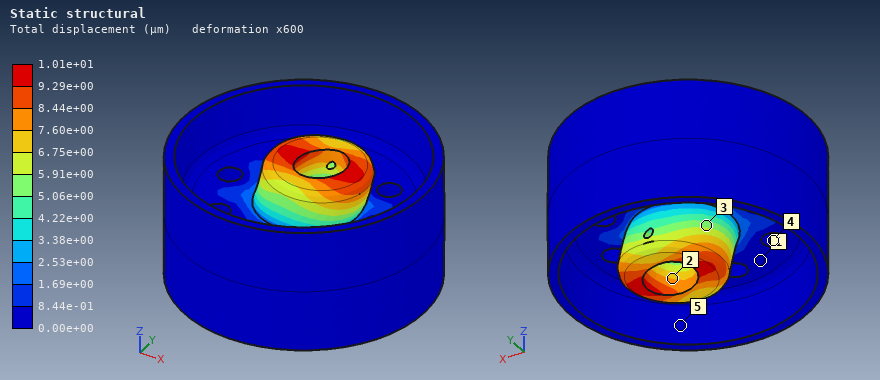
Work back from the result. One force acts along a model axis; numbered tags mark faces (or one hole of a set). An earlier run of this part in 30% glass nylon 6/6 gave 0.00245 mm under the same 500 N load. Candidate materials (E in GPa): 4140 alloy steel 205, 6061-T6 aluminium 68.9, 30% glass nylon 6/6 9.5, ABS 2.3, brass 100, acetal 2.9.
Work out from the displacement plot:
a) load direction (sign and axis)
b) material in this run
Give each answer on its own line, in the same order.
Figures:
+X
ABS
